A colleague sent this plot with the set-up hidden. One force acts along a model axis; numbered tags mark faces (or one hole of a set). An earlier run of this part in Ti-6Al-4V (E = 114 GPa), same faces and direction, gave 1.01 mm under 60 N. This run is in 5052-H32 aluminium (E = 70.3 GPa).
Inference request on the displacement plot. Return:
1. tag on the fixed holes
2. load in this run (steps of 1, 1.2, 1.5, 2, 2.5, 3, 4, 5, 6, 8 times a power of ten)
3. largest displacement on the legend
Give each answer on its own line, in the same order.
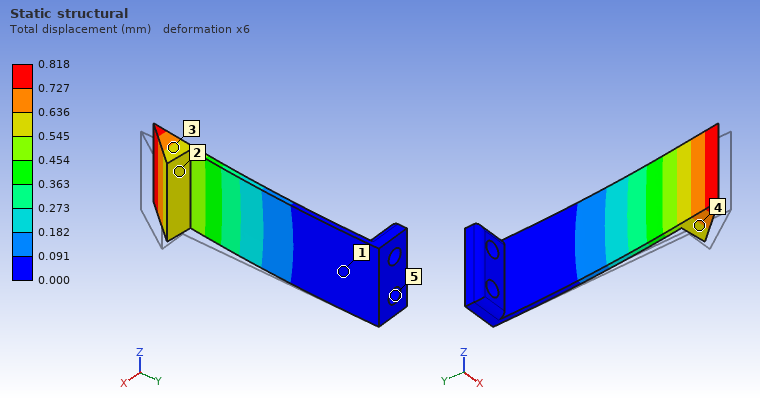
5
30 N
0.818 mm
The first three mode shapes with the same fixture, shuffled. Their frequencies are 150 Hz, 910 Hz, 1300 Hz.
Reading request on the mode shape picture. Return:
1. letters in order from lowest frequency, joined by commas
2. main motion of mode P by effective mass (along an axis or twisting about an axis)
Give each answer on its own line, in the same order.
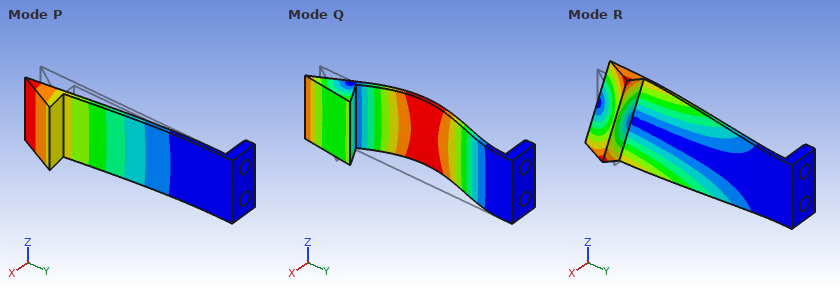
P, R, Q
along X
